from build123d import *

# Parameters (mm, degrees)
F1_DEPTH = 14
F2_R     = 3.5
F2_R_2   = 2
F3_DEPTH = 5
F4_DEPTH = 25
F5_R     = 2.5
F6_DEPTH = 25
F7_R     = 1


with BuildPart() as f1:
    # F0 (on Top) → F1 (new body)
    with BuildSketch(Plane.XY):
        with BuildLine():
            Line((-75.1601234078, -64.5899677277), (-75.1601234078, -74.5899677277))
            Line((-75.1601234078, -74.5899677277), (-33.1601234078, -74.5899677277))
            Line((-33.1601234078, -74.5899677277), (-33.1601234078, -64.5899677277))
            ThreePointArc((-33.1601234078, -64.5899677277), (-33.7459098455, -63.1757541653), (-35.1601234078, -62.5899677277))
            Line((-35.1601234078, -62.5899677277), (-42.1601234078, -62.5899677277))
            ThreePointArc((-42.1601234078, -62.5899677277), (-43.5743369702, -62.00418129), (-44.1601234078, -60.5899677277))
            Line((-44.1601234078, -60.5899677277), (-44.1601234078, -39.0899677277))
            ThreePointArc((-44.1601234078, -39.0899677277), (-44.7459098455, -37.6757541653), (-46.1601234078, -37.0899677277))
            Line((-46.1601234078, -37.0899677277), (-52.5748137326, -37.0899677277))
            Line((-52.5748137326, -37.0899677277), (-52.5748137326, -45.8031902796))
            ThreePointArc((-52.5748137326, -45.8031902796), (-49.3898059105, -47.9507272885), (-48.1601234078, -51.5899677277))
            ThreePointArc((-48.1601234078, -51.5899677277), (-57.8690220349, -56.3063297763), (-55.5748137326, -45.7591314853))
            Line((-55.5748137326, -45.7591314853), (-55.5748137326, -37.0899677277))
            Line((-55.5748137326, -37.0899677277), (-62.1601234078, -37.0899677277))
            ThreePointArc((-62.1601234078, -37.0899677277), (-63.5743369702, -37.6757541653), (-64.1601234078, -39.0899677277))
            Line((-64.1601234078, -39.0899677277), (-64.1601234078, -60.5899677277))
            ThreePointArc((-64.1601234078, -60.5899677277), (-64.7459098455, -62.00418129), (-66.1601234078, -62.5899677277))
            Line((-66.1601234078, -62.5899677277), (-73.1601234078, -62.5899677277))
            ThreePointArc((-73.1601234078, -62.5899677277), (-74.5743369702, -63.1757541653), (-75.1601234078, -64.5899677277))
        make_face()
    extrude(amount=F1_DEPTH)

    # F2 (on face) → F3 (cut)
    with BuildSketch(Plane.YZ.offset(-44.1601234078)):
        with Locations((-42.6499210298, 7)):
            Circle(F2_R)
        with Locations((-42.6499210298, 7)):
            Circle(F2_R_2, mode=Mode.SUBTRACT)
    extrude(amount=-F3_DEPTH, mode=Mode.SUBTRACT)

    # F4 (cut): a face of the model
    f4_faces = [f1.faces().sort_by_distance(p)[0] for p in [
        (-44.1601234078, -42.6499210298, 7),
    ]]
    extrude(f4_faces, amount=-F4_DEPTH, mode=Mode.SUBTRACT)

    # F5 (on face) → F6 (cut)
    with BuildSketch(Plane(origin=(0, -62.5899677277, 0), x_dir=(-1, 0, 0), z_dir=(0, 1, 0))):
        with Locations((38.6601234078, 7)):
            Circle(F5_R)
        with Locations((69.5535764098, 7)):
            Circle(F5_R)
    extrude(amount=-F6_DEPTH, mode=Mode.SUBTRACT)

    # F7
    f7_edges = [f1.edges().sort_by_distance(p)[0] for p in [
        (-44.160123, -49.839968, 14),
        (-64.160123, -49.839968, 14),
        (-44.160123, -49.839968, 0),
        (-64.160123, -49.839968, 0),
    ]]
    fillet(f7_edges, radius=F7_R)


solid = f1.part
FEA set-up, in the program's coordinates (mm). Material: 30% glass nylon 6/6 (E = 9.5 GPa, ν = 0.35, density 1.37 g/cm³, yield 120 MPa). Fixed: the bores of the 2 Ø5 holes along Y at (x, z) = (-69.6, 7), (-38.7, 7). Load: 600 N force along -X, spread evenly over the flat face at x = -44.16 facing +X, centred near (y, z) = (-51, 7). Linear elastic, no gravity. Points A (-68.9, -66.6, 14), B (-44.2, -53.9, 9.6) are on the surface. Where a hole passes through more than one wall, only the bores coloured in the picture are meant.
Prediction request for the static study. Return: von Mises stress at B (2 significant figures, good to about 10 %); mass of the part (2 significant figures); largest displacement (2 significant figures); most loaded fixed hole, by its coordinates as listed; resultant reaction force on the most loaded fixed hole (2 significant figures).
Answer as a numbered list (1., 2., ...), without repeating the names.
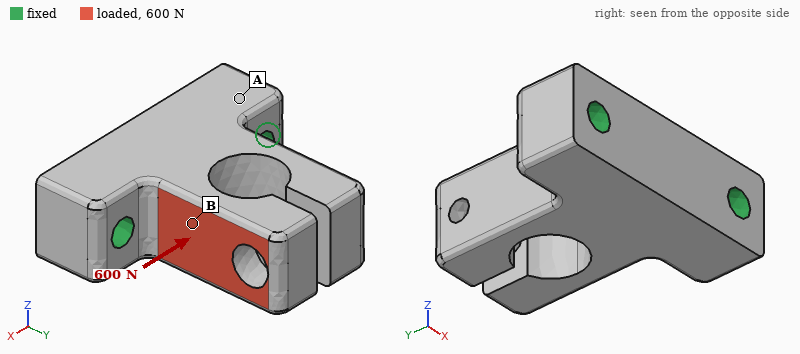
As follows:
1. 47 MPa
2. 16 g
3. 0.47 mm
4. (-69.6, 7)
5. 510 N
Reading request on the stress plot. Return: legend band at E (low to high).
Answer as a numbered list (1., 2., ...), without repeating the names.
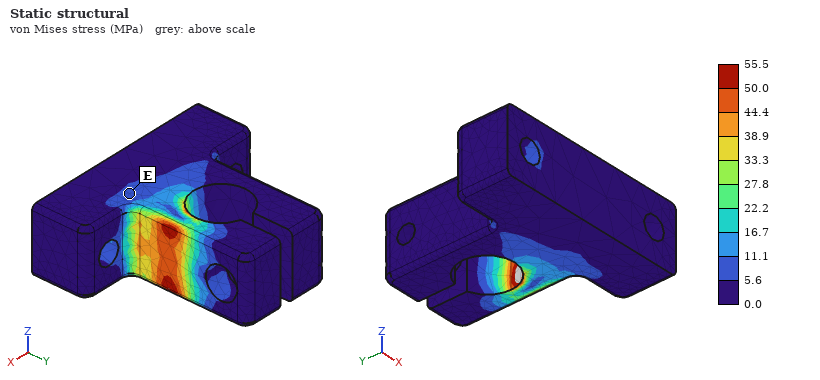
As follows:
1. 5.6 to 11.1 MPa
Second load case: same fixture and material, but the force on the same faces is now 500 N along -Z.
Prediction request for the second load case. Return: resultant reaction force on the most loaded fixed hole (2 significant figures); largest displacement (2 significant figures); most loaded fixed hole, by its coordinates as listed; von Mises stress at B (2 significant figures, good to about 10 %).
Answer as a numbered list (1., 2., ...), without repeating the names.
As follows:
1. 430 N
2. 0.21 mm
3. (-38.7, 7)
4. 17 MPa
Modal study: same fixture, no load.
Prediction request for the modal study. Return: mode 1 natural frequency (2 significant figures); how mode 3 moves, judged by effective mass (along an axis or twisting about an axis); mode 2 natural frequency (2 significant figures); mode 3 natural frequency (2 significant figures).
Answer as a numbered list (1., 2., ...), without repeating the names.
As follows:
1. 3200 Hz
2. along Z
3. 3400 Hz
4. 4200 Hz
